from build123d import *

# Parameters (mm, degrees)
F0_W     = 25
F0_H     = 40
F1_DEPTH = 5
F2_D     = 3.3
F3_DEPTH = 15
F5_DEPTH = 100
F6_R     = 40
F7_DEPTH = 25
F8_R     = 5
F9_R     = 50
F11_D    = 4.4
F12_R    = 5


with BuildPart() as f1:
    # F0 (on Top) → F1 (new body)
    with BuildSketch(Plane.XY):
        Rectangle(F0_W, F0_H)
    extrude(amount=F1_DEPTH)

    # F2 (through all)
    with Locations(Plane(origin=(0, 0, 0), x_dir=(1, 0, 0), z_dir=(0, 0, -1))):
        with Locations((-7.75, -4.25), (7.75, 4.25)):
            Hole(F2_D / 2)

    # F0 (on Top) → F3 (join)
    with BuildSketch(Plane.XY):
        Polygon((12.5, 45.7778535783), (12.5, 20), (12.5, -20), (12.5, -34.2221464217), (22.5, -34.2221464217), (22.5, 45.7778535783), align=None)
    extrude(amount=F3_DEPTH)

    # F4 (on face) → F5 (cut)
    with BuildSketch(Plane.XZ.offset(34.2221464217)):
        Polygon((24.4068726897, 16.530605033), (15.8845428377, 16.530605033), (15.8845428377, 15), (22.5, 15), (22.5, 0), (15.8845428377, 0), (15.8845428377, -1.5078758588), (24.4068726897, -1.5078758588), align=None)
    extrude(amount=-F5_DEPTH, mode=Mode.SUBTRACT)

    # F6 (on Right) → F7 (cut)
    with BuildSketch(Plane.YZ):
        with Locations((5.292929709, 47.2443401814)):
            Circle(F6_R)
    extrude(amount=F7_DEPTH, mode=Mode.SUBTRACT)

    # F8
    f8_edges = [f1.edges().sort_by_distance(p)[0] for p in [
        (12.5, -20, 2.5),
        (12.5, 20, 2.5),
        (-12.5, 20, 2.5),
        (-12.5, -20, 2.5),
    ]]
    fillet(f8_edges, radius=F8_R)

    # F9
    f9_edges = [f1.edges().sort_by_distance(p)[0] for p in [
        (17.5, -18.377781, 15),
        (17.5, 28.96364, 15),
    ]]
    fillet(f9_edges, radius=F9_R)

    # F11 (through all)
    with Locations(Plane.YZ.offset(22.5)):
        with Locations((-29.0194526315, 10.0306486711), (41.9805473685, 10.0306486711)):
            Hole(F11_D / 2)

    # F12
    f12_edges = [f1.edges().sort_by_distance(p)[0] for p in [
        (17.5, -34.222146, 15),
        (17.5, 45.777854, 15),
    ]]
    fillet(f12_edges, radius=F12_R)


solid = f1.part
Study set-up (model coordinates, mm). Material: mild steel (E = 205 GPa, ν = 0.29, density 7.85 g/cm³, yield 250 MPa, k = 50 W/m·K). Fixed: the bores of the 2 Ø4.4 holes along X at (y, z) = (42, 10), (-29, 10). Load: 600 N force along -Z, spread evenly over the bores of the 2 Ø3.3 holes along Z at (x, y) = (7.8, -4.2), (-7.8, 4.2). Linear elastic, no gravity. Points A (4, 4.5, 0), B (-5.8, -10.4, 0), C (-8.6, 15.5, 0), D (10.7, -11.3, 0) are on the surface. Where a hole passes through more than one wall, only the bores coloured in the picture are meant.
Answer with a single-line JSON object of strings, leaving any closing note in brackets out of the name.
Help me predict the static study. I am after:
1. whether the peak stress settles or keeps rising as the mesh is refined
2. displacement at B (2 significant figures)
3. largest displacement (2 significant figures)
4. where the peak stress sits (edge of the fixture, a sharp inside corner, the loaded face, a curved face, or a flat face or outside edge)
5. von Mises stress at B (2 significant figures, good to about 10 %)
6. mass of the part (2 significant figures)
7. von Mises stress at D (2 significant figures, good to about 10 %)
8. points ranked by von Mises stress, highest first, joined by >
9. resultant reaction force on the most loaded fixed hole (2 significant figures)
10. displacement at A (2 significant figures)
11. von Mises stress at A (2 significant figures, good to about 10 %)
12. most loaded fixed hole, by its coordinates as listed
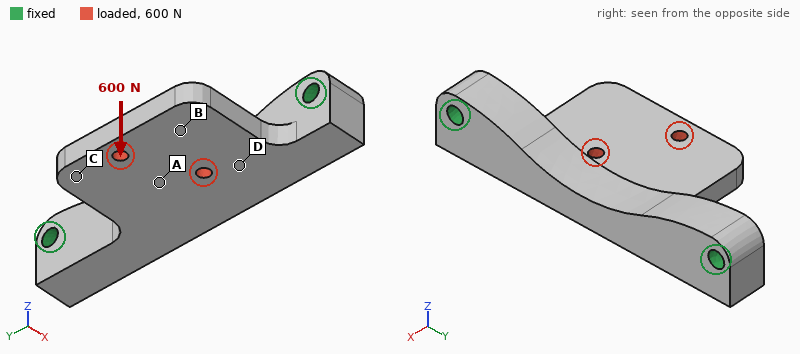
{"whether the peak stress settles or keeps rising as the mesh is refined": "keeps rising", "displacement at B": "29 µm", "largest displacement": "46 µm", "where the peak stress sits": "edge of the fixture", "von Mises stress at B": "11 MPa", "mass of the part": "110 g", "von Mises stress at D": "37 MPa", "points ranked by von Mises stress, highest first, joined by >": "D > A > B > C", "resultant reaction force on the most loaded fixed hole": "600 N", "displacement at A": "19 µm", "von Mises stress at A": "26 MPa", "most loaded fixed hole, by its coordinates as listed": "(-29, 10)"}
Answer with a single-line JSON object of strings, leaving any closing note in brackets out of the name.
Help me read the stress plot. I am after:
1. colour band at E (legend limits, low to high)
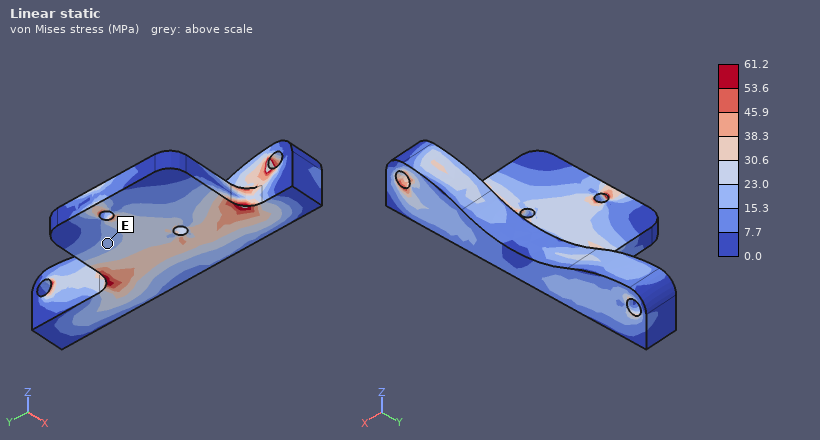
{"colour band at E": "15.3 to 23.0 MPa"}
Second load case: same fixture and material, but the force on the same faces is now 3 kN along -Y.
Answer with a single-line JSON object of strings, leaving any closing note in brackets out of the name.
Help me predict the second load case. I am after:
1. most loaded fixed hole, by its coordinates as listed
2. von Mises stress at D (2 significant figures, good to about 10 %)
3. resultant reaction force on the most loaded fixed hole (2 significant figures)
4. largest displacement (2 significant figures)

{"most loaded fixed hole, by its coordinates as listed": "(-29, 10)", "von Mises stress at D": "18 MPa", "resultant reaction force on the most loaded fixed hole": "1.9 kN", "largest displacement": "17 µm"}
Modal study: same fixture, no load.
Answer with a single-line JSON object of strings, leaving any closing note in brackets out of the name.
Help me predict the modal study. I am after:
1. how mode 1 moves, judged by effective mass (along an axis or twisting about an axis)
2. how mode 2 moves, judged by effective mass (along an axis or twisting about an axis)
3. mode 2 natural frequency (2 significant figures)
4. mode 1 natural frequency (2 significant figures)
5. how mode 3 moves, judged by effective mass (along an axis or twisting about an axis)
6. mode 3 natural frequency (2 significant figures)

{"how mode 1 moves, judged by effective mass": "along Z", "how mode 2 moves, judged by effective mass": "along X", "mode 2 natural frequency": "8500 Hz", "mode 1 natural frequency": "3800 Hz", "how mode 3 moves, judged by effective mass": "along X", "mode 3 natural frequency": "9100 Hz"}
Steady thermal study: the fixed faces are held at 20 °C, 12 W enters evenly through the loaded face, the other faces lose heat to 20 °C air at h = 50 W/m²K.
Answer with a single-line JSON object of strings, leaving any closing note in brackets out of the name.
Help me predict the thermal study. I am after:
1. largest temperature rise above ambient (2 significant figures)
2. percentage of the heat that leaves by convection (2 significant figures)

{"largest temperature rise above ambient": "35 K", "percentage of the heat that leaves by convection": "33 %"}
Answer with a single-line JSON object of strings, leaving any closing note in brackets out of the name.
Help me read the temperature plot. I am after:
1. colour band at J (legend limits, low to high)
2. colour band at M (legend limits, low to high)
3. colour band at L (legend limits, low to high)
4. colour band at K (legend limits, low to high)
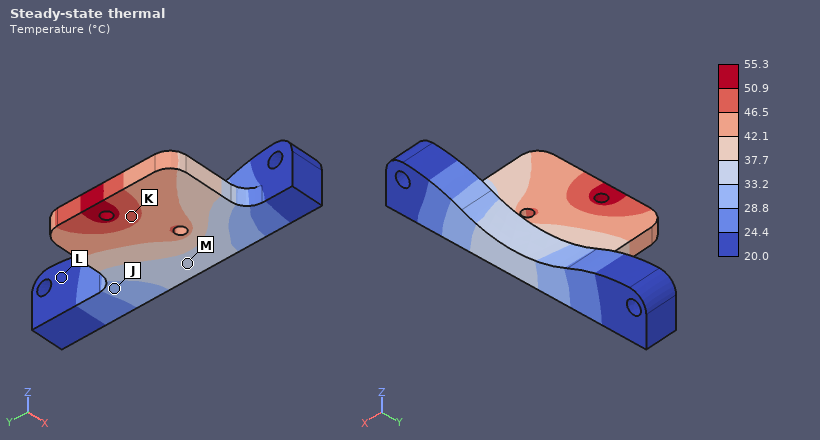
{"colour band at J": "28.8 to 33.2 °C", "colour band at M": "33.2 to 37.7 °C", "colour band at L": "20.0 to 24.4 °C", "colour band at K": "46.5 to 50.9 °C"}
